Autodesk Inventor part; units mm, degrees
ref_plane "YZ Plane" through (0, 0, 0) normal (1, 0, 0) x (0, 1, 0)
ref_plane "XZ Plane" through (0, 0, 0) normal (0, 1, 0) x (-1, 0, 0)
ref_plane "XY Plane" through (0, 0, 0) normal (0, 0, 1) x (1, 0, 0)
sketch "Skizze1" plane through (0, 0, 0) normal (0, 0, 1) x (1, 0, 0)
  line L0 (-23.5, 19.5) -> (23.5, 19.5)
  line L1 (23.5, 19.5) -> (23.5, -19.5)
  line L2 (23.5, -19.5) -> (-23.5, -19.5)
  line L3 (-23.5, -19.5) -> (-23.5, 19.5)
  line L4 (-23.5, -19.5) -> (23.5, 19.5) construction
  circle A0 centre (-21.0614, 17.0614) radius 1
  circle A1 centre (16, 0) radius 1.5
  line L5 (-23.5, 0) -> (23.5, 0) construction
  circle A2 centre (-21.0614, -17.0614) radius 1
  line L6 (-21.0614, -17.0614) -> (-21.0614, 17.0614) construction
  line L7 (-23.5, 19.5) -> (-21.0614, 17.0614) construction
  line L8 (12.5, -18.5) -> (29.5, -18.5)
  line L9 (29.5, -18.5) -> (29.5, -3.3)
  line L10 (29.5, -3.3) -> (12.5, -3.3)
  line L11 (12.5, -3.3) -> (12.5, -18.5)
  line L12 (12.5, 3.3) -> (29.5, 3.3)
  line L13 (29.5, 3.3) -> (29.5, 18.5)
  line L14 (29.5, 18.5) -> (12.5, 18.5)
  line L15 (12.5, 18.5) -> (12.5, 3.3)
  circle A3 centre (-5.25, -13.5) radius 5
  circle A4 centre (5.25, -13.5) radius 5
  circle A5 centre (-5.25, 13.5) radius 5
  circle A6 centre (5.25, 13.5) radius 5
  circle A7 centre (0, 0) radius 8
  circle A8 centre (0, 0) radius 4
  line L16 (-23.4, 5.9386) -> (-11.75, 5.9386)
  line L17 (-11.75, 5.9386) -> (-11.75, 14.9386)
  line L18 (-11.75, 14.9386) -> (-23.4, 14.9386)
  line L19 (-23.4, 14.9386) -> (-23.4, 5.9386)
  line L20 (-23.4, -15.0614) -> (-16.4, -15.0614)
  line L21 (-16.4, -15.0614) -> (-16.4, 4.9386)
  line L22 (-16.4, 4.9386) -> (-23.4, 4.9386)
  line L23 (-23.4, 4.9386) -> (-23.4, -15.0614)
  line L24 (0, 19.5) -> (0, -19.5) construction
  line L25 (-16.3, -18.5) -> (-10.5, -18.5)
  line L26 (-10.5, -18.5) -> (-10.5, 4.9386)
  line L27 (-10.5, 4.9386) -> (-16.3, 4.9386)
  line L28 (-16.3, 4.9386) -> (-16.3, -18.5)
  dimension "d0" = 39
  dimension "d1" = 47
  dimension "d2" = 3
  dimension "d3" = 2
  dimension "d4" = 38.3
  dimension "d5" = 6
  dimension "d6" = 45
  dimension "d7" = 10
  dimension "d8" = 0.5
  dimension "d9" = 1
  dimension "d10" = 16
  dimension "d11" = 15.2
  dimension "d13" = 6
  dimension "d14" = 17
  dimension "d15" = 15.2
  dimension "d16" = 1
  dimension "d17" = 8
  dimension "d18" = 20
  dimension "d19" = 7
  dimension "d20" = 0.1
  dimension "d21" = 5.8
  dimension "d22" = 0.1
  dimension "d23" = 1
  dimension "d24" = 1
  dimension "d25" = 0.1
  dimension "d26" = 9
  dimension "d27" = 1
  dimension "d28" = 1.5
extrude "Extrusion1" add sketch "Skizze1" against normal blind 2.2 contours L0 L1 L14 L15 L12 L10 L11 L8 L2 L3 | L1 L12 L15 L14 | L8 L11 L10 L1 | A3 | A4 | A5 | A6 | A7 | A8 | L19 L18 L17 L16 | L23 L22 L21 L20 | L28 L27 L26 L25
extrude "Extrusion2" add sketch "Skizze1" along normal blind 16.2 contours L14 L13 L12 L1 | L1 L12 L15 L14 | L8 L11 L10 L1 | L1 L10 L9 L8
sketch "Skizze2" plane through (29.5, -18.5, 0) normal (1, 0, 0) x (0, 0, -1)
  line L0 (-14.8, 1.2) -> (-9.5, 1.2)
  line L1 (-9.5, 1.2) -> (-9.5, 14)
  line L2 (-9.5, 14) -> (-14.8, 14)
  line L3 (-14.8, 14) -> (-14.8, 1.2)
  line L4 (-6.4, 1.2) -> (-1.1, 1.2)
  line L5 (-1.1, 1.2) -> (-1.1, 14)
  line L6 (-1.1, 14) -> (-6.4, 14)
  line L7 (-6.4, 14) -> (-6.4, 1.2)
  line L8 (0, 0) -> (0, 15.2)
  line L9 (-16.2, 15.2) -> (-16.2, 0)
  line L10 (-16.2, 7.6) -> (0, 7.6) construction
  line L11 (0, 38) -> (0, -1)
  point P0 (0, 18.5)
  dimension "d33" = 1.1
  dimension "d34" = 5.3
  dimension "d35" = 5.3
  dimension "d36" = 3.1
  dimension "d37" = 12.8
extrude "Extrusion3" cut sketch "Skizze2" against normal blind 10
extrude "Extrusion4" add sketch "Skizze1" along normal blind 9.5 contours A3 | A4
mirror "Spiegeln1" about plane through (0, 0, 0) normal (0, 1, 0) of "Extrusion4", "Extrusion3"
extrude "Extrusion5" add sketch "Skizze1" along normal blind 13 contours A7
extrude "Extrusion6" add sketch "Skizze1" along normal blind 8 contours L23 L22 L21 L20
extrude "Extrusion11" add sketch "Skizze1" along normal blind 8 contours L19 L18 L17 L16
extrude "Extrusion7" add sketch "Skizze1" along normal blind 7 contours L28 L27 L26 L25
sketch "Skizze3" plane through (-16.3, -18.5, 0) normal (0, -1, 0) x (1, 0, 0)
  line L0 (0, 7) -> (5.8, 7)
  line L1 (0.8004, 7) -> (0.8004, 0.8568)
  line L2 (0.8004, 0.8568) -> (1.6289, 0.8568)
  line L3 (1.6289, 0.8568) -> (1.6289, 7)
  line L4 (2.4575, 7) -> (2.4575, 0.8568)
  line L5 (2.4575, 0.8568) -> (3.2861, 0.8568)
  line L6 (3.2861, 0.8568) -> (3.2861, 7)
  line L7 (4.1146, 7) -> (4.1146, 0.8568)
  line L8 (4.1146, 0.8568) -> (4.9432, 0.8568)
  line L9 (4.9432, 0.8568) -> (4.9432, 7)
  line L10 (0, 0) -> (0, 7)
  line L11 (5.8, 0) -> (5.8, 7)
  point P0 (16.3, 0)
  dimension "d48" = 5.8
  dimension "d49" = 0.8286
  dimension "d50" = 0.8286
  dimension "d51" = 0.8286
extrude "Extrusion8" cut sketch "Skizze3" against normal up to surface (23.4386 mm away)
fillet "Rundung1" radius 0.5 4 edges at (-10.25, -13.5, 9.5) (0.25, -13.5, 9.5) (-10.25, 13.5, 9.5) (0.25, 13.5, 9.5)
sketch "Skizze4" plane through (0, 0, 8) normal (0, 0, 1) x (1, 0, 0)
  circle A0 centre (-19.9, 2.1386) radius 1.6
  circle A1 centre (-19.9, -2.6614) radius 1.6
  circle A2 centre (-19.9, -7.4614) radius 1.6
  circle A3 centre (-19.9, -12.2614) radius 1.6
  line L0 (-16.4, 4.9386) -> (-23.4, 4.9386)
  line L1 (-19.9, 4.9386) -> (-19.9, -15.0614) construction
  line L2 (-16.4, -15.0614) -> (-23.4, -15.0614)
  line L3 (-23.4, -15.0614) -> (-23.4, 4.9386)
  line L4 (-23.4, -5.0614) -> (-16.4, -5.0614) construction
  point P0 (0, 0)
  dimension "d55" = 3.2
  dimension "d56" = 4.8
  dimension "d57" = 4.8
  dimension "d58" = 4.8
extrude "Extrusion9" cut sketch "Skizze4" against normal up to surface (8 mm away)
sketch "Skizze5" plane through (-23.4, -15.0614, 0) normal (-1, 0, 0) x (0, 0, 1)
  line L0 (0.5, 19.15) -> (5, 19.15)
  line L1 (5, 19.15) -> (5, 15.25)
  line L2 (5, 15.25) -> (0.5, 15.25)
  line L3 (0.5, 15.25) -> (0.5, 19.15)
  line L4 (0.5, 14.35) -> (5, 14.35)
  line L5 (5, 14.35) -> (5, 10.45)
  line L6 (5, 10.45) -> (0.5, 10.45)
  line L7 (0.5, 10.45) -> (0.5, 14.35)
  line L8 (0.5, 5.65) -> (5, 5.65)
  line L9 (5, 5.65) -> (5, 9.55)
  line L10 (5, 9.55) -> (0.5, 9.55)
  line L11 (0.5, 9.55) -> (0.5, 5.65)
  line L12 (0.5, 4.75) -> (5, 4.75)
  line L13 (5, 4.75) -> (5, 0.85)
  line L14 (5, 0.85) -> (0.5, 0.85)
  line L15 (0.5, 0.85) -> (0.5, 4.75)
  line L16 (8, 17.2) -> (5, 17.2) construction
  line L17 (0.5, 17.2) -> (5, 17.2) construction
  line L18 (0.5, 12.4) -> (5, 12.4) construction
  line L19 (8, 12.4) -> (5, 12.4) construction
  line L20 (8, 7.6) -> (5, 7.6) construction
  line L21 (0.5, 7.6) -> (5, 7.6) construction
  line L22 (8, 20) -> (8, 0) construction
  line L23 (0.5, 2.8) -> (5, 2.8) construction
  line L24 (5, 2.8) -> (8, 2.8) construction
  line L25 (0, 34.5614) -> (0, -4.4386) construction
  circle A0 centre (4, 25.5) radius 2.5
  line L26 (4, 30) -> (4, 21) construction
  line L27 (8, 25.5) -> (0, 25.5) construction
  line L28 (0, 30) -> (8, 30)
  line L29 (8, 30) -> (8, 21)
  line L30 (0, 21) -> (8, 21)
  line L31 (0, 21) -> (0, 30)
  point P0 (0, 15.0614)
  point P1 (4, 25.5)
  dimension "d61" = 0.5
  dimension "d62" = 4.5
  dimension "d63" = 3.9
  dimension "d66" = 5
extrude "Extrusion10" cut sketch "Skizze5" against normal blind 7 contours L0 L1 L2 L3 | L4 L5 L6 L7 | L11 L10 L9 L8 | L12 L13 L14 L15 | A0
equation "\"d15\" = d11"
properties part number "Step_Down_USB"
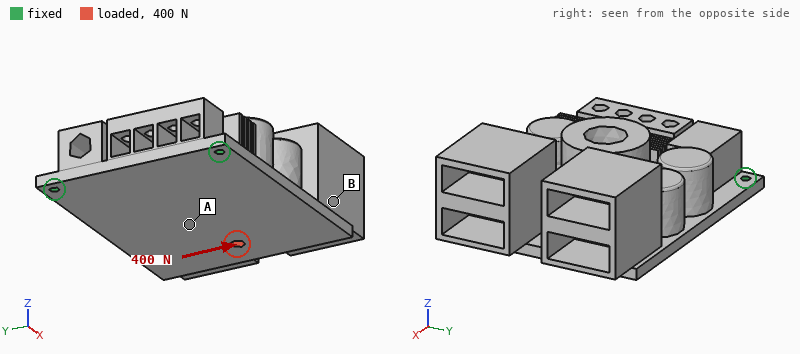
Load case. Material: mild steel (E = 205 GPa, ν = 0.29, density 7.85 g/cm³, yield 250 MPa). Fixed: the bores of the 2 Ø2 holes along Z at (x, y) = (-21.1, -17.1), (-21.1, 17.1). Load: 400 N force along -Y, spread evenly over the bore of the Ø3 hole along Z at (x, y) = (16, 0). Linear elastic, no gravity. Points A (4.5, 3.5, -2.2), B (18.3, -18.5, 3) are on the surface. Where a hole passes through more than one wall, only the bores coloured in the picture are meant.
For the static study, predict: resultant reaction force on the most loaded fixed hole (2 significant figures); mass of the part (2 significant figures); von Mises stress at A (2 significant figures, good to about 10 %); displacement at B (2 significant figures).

480 N
130 g
9.6 MPa
6.2 µm
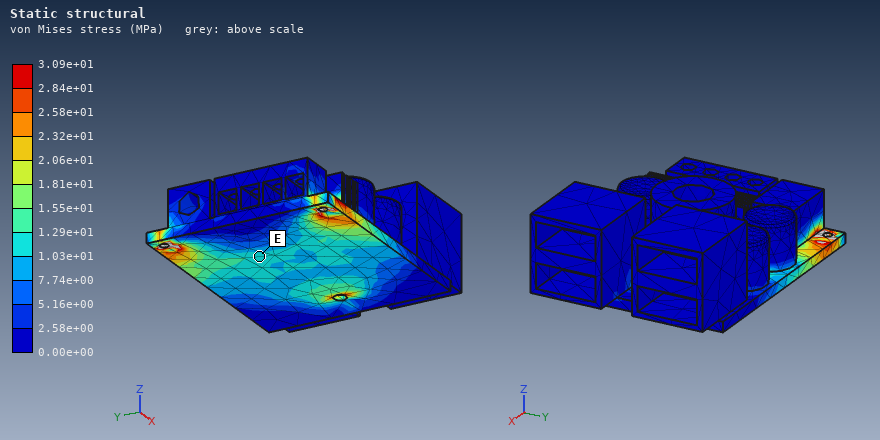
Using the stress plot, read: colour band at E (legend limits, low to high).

1.03e+01 to 1.29e+01 MPa
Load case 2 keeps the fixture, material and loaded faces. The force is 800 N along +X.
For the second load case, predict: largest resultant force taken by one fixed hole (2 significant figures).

420 N
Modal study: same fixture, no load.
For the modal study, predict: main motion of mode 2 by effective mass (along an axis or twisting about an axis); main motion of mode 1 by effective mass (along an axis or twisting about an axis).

along Y
along Z
